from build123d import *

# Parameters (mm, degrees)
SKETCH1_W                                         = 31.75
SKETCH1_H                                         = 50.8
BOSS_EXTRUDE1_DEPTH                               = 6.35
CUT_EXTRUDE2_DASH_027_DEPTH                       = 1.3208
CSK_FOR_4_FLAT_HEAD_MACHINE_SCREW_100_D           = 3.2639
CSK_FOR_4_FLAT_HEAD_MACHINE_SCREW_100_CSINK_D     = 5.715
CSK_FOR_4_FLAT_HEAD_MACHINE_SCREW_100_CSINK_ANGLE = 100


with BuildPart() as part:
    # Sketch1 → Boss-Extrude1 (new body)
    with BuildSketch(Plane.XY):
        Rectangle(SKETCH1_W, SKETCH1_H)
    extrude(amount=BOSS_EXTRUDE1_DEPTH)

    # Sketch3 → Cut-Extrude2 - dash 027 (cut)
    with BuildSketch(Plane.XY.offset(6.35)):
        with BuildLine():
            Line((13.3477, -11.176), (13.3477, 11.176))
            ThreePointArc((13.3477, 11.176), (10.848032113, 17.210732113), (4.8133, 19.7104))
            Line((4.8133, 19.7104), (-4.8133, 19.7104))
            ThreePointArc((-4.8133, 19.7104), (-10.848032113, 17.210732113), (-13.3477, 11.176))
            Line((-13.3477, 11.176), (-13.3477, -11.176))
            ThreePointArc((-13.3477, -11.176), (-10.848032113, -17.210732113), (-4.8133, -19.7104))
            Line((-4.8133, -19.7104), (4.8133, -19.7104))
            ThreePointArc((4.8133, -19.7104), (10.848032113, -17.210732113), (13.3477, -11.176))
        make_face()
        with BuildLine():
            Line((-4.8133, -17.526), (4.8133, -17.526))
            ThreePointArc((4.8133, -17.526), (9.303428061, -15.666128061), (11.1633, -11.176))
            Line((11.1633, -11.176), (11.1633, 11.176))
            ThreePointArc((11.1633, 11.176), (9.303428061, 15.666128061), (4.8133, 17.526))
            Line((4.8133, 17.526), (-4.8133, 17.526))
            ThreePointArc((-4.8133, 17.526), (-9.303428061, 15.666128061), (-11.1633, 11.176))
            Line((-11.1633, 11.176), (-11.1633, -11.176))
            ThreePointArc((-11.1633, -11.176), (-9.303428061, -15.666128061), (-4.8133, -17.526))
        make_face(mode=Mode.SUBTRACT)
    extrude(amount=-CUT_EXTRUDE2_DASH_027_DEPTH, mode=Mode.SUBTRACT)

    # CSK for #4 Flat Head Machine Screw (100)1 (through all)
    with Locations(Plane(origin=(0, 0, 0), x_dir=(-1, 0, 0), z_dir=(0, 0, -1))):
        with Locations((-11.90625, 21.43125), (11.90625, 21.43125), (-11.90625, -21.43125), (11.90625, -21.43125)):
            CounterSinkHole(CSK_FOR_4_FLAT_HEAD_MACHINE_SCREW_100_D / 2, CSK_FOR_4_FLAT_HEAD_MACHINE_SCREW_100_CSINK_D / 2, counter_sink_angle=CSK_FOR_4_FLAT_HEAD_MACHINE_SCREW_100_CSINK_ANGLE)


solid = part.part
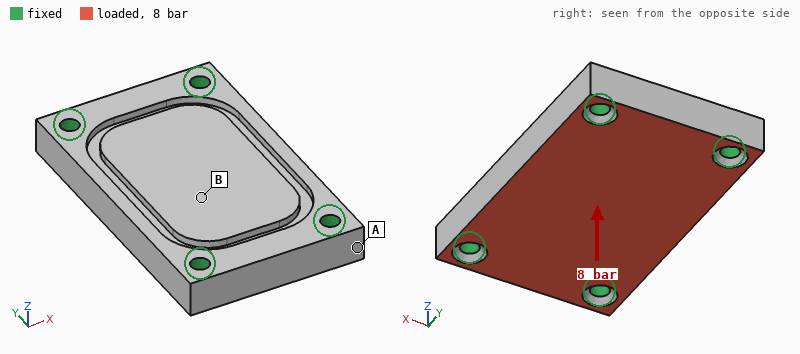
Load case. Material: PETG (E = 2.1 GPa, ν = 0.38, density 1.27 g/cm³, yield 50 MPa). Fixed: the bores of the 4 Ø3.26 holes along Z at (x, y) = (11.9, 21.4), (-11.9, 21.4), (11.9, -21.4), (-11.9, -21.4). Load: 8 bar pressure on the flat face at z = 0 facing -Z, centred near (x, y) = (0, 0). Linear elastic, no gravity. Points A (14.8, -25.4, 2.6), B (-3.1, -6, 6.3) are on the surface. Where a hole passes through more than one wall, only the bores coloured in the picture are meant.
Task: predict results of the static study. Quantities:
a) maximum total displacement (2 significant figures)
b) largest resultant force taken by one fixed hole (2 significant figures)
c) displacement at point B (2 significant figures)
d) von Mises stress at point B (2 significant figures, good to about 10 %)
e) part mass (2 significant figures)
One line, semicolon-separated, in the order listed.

0.30 mm; 310 N; 0.25 mm; 8.6 MPa; 12 g
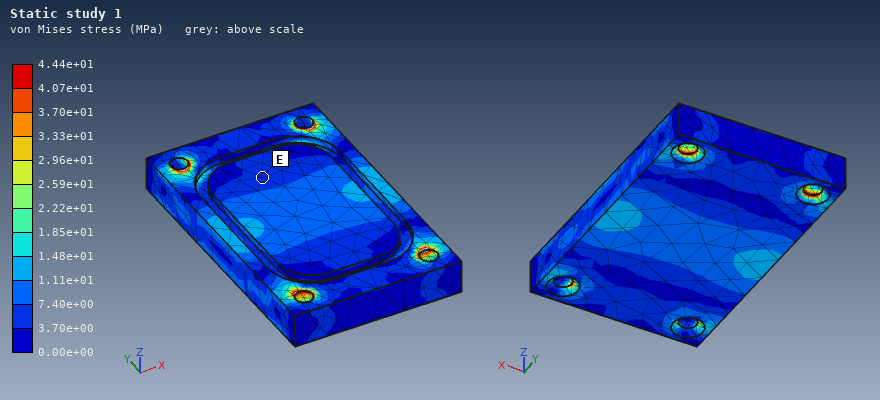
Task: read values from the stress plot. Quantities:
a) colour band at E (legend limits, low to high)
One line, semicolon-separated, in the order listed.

3.70e+00 to 7.40e+00 MPa
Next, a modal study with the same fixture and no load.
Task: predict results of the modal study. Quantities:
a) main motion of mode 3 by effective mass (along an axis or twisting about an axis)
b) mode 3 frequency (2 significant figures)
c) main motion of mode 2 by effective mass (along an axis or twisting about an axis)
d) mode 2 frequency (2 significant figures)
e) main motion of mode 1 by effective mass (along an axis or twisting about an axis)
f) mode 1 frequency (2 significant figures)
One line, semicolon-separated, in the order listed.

along X; 7400 Hz; twisting about Y; 4900 Hz; along Z; 3400 Hz
